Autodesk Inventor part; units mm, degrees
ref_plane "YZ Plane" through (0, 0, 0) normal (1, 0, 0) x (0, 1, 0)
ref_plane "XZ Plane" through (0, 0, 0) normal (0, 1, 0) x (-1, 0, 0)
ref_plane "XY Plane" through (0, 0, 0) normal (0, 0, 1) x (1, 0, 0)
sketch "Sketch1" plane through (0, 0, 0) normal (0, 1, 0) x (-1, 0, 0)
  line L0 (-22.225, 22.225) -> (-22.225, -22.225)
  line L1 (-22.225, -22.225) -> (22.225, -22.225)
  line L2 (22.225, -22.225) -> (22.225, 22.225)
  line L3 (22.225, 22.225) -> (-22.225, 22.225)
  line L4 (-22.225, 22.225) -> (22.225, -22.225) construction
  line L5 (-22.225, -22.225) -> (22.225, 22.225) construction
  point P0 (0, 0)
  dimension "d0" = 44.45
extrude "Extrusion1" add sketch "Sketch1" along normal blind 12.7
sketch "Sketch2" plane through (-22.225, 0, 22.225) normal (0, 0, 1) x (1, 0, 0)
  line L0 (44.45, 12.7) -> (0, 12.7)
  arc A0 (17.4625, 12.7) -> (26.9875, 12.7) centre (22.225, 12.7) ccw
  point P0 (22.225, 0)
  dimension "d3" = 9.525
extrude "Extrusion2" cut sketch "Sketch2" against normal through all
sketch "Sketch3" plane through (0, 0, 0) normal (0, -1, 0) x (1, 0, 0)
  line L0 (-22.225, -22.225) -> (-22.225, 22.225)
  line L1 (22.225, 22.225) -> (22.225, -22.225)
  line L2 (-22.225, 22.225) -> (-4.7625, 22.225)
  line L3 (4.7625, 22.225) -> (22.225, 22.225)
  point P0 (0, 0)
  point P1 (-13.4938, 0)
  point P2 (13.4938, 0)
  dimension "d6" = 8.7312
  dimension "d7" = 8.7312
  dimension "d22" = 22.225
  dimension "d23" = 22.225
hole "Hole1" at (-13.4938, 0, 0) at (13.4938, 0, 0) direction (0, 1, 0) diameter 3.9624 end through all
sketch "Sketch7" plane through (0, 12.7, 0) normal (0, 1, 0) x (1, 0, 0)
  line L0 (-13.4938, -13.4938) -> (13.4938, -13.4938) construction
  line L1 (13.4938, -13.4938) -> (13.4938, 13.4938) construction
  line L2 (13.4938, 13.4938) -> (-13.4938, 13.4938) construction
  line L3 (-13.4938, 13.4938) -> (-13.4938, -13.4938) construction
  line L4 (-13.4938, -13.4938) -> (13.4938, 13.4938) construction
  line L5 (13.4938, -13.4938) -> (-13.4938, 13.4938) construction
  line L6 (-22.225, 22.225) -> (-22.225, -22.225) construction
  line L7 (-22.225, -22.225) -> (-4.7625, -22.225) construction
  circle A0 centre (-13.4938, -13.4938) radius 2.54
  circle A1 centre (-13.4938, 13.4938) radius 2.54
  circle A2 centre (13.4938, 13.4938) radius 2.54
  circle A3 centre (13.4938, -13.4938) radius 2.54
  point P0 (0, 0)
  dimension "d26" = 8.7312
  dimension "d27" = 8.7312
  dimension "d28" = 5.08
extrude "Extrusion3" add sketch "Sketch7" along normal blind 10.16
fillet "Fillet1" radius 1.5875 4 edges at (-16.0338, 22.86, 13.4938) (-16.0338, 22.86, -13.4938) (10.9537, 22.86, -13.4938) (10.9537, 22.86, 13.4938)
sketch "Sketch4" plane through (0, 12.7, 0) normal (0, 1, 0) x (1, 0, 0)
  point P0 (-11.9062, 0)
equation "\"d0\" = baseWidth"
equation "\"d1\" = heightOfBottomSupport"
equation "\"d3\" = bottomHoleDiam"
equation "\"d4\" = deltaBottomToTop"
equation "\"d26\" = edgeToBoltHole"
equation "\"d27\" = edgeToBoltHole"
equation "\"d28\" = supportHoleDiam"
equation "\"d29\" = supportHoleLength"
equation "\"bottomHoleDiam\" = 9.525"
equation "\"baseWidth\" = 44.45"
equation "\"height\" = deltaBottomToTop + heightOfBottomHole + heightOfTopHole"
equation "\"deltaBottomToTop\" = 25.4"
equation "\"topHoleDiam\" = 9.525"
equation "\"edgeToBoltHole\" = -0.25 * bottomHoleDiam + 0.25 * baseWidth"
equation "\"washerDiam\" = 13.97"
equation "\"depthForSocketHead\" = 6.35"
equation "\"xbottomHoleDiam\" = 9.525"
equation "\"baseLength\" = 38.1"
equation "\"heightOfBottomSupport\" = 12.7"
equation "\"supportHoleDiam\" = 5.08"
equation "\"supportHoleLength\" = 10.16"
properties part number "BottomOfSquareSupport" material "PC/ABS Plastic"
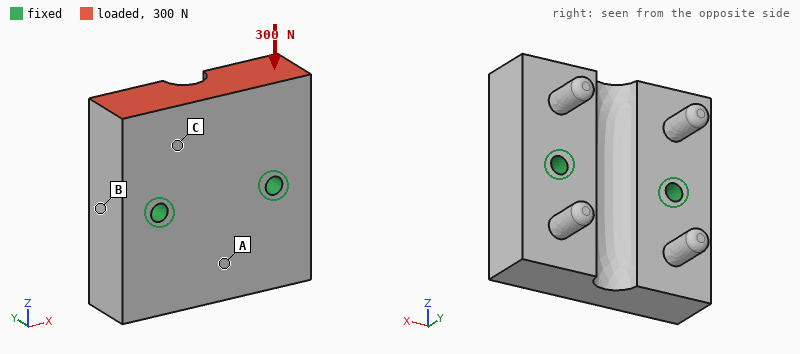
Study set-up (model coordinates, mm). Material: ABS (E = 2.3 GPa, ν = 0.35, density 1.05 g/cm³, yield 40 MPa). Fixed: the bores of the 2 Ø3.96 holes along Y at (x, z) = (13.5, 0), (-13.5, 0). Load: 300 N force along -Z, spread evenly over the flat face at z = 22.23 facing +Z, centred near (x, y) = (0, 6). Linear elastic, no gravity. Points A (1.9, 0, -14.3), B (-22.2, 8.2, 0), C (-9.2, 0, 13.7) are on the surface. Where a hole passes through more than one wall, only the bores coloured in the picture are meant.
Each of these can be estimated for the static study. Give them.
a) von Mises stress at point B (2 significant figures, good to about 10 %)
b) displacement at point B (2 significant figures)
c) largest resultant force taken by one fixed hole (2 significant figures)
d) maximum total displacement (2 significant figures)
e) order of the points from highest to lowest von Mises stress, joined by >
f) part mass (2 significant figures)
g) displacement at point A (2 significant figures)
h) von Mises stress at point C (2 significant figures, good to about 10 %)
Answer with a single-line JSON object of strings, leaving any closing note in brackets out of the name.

{"von Mises stress at point B": "0.34 MPa", "displacement at point B": "2.2 µm", "largest resultant force taken by one fixed hole": "150 N", "maximum total displacement": "7.2 µm", "order of the points from highest to lowest von Mises stress, joined by >": "C > B > A", "part mass": "25 g", "displacement at point A": "2.0 µm", "von Mises stress at point C": "0.60 MPa"}
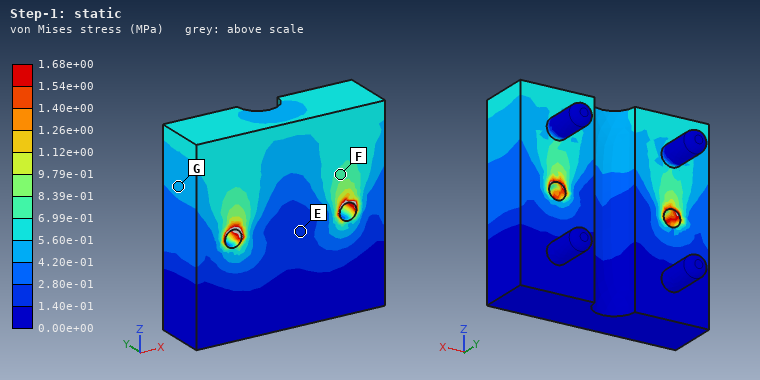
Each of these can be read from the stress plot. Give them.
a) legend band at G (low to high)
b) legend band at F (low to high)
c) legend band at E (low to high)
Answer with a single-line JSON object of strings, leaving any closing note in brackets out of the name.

{"legend band at G": "4.20e-01 to 5.60e-01 MPa", "legend band at F": "6.99e-01 to 8.39e-01 MPa", "legend band at E": "1.40e-01 to 2.80e-01 MPa"}
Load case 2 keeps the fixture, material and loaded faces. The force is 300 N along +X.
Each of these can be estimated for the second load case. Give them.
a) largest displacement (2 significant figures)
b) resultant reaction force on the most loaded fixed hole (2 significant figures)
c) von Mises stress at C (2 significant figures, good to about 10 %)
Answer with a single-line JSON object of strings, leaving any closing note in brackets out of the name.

{"largest displacement": "40 µm", "resultant reaction force on the most loaded fixed hole": "270 N", "von Mises stress at C": "1.3 MPa"}
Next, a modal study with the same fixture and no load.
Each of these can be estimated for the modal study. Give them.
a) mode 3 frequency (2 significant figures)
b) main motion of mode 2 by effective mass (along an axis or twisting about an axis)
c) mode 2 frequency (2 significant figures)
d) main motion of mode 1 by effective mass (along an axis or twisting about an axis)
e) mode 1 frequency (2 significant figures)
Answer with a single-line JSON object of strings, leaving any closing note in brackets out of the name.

{"mode 3 frequency": "5300 Hz", "main motion of mode 2 by effective mass": "along Y", "mode 2 frequency": "4900 Hz", "main motion of mode 1 by effective mass": "twisting about X", "mode 1 frequency": "3700 Hz"}
